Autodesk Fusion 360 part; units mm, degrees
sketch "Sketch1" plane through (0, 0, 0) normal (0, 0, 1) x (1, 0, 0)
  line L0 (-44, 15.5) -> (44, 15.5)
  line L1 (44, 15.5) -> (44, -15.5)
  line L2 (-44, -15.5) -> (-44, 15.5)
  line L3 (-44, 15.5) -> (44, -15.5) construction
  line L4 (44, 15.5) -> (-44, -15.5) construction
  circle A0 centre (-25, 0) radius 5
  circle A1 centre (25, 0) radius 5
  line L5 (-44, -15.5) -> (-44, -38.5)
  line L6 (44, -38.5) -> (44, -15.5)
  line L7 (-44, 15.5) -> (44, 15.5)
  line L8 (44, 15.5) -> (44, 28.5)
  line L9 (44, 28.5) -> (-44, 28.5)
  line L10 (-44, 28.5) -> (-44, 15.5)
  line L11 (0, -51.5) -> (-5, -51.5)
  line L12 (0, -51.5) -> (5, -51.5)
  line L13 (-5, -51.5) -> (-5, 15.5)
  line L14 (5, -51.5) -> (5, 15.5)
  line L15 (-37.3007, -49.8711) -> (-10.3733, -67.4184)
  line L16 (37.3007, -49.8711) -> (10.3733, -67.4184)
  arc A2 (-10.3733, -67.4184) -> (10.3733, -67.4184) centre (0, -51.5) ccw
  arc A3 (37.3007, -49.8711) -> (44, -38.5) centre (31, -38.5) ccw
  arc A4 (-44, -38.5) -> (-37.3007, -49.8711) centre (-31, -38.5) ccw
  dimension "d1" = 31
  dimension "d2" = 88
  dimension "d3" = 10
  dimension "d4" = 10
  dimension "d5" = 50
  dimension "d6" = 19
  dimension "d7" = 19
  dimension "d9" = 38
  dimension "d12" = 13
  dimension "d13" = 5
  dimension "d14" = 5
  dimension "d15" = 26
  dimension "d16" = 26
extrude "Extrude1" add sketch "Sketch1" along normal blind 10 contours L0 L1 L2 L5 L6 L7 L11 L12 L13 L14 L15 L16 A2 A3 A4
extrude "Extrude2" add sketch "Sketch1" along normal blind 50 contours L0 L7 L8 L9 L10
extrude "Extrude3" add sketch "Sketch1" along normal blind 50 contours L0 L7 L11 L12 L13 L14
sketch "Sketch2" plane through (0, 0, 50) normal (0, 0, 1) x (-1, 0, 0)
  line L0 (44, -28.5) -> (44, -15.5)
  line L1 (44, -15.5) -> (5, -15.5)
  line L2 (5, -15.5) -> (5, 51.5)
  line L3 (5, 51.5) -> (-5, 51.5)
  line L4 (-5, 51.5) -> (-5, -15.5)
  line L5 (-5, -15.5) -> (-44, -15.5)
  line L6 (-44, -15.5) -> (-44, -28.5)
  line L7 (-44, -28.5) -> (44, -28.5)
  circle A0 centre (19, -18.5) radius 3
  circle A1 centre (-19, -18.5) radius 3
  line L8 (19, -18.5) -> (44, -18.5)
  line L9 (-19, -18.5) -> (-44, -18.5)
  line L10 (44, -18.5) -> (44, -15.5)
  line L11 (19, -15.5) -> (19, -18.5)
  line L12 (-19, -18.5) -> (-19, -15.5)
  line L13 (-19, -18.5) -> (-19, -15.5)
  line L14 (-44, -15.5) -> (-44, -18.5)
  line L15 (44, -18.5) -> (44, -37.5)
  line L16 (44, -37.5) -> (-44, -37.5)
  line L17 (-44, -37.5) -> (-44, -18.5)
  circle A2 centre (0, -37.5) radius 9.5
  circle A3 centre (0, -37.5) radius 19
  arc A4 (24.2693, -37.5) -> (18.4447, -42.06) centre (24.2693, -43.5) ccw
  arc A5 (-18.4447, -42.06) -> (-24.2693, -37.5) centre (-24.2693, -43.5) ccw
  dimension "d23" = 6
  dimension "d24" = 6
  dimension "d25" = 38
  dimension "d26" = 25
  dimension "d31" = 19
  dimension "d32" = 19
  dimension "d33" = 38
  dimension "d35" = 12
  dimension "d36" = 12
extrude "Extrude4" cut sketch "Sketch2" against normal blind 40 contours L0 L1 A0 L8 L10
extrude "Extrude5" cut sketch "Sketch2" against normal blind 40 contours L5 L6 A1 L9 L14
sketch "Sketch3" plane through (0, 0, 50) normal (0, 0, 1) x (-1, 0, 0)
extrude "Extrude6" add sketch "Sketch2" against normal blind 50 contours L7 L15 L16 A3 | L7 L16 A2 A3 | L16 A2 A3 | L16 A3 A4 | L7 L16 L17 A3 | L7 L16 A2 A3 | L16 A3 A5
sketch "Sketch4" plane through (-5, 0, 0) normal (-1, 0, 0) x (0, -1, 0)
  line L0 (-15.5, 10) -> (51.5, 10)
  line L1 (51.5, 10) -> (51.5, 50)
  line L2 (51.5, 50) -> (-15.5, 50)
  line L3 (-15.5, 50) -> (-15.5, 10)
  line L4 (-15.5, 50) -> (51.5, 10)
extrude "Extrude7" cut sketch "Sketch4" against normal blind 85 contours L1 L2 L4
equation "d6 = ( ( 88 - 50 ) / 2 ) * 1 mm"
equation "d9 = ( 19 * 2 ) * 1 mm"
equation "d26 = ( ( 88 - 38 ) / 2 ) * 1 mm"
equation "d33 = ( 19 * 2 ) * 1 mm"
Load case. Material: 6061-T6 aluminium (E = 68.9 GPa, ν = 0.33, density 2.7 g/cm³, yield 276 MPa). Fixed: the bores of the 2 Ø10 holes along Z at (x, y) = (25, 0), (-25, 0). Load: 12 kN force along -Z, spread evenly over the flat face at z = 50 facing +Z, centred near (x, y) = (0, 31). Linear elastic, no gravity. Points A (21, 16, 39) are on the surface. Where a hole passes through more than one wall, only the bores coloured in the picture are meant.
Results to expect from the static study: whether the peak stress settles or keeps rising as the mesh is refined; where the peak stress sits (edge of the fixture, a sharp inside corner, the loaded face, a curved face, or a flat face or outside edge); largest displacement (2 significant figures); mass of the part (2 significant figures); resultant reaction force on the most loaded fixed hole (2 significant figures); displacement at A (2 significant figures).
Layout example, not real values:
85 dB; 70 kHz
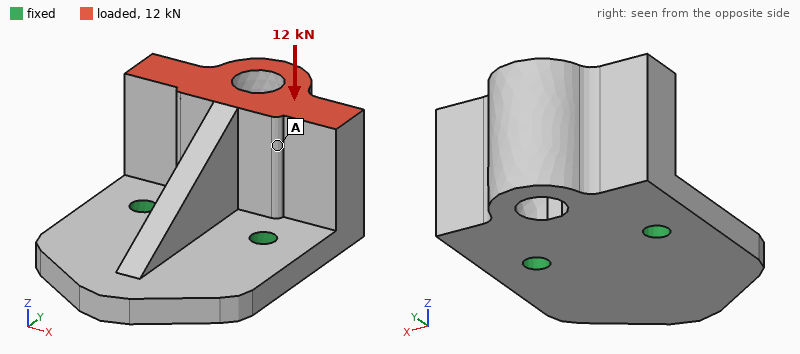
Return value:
keeps rising; edge of the fixture; 0.34 mm; 500 g; 6.1 kN; 0.17 mm
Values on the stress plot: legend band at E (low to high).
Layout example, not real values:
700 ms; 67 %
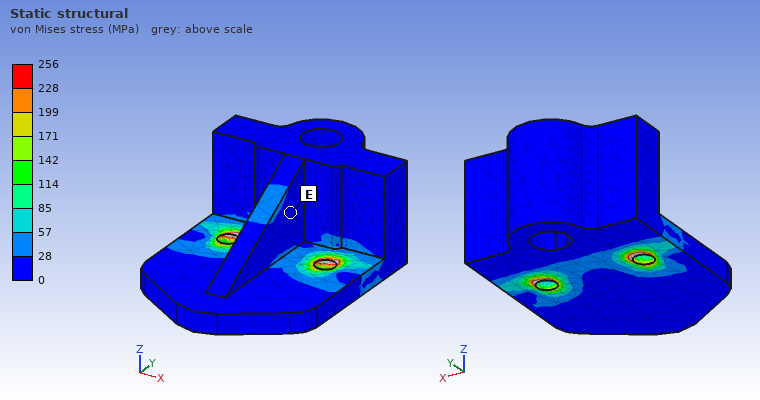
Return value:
0 to 28 MPa
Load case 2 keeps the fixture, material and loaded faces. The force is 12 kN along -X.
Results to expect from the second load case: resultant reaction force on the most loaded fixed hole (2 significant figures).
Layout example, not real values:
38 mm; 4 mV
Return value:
13 kN
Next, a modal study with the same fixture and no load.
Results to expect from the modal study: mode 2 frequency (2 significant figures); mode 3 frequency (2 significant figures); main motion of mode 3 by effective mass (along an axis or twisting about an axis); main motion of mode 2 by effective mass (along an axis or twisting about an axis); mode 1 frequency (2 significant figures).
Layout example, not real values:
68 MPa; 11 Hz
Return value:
3900 Hz; 4200 Hz; along Z; along X; 1700 Hz
